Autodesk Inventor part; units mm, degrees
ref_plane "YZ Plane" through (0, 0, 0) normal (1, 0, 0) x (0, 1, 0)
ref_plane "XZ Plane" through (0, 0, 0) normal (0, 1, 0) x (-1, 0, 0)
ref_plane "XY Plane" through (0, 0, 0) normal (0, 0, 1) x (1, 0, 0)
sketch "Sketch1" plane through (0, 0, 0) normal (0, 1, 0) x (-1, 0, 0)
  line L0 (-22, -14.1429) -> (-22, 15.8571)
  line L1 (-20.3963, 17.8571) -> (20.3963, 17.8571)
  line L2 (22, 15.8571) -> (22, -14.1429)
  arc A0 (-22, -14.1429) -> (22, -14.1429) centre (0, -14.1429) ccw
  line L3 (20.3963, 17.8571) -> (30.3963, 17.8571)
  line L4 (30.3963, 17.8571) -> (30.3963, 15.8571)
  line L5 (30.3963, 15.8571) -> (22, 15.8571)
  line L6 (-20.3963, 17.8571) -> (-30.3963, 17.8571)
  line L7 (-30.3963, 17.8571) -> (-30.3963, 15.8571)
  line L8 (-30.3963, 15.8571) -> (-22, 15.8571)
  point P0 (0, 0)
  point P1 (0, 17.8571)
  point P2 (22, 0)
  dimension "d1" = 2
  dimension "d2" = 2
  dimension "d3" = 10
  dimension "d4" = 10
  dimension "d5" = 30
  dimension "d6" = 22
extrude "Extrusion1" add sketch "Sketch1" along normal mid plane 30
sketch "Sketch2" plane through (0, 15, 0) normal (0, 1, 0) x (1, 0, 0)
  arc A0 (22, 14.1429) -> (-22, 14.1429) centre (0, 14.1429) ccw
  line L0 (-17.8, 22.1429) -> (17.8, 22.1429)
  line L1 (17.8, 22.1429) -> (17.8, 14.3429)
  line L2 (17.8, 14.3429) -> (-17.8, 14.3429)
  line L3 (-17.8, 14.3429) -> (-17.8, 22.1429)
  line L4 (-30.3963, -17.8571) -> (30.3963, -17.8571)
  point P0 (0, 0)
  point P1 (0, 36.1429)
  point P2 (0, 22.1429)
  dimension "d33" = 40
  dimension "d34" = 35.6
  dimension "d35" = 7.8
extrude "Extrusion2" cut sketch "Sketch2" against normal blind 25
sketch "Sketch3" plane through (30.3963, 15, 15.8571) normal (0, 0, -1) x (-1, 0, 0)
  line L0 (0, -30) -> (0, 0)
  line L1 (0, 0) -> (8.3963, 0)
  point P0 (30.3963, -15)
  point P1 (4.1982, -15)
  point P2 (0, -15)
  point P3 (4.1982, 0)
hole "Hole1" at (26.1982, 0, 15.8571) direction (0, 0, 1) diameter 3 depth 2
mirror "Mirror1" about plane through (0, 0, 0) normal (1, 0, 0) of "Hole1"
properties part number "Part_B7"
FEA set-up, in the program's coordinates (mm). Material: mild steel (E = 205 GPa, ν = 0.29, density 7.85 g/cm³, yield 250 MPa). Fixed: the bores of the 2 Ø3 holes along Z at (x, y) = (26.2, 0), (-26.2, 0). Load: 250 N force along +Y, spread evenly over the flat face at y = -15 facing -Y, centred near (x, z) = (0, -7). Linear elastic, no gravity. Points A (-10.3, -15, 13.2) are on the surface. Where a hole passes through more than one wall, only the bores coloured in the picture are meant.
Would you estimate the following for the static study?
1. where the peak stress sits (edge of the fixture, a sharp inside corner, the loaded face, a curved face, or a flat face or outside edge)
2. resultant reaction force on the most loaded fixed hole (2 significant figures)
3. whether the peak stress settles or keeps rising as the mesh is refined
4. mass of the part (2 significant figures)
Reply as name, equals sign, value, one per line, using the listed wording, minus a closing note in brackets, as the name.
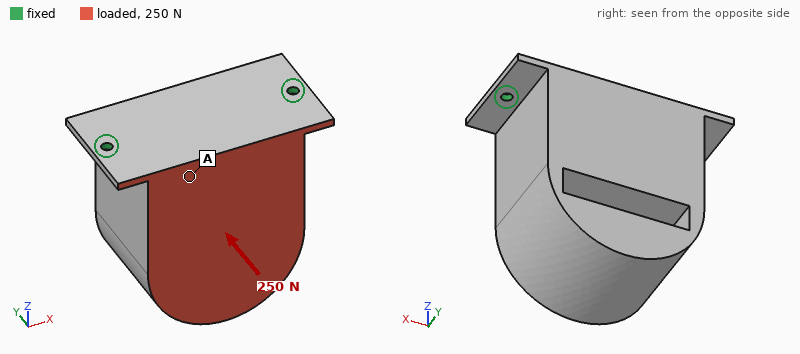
where the peak stress sits = edge of the fixture
resultant reaction force on the most loaded fixed hole = 130 N
whether the peak stress settles or keeps rising as the mesh is refined = keeps rising
mass of the part = 460 g
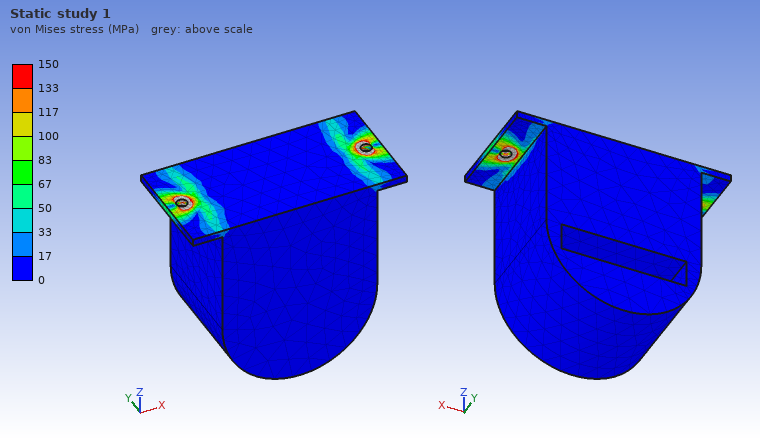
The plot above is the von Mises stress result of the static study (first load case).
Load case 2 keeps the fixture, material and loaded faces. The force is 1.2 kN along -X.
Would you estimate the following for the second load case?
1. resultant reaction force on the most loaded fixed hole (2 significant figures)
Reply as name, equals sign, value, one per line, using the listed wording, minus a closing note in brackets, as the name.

resultant reaction force on the most loaded fixed hole = 910 N
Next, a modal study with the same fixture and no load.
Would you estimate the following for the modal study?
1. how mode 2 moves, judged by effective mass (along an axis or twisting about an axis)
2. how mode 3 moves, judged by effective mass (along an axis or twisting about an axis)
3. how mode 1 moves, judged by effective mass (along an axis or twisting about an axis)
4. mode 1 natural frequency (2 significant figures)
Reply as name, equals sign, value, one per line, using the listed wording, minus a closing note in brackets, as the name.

how mode 2 moves, judged by effective mass = along X
how mode 3 moves, judged by effective mass = along Z
how mode 1 moves, judged by effective mass = along Y
mode 1 natural frequency = 390 Hz
